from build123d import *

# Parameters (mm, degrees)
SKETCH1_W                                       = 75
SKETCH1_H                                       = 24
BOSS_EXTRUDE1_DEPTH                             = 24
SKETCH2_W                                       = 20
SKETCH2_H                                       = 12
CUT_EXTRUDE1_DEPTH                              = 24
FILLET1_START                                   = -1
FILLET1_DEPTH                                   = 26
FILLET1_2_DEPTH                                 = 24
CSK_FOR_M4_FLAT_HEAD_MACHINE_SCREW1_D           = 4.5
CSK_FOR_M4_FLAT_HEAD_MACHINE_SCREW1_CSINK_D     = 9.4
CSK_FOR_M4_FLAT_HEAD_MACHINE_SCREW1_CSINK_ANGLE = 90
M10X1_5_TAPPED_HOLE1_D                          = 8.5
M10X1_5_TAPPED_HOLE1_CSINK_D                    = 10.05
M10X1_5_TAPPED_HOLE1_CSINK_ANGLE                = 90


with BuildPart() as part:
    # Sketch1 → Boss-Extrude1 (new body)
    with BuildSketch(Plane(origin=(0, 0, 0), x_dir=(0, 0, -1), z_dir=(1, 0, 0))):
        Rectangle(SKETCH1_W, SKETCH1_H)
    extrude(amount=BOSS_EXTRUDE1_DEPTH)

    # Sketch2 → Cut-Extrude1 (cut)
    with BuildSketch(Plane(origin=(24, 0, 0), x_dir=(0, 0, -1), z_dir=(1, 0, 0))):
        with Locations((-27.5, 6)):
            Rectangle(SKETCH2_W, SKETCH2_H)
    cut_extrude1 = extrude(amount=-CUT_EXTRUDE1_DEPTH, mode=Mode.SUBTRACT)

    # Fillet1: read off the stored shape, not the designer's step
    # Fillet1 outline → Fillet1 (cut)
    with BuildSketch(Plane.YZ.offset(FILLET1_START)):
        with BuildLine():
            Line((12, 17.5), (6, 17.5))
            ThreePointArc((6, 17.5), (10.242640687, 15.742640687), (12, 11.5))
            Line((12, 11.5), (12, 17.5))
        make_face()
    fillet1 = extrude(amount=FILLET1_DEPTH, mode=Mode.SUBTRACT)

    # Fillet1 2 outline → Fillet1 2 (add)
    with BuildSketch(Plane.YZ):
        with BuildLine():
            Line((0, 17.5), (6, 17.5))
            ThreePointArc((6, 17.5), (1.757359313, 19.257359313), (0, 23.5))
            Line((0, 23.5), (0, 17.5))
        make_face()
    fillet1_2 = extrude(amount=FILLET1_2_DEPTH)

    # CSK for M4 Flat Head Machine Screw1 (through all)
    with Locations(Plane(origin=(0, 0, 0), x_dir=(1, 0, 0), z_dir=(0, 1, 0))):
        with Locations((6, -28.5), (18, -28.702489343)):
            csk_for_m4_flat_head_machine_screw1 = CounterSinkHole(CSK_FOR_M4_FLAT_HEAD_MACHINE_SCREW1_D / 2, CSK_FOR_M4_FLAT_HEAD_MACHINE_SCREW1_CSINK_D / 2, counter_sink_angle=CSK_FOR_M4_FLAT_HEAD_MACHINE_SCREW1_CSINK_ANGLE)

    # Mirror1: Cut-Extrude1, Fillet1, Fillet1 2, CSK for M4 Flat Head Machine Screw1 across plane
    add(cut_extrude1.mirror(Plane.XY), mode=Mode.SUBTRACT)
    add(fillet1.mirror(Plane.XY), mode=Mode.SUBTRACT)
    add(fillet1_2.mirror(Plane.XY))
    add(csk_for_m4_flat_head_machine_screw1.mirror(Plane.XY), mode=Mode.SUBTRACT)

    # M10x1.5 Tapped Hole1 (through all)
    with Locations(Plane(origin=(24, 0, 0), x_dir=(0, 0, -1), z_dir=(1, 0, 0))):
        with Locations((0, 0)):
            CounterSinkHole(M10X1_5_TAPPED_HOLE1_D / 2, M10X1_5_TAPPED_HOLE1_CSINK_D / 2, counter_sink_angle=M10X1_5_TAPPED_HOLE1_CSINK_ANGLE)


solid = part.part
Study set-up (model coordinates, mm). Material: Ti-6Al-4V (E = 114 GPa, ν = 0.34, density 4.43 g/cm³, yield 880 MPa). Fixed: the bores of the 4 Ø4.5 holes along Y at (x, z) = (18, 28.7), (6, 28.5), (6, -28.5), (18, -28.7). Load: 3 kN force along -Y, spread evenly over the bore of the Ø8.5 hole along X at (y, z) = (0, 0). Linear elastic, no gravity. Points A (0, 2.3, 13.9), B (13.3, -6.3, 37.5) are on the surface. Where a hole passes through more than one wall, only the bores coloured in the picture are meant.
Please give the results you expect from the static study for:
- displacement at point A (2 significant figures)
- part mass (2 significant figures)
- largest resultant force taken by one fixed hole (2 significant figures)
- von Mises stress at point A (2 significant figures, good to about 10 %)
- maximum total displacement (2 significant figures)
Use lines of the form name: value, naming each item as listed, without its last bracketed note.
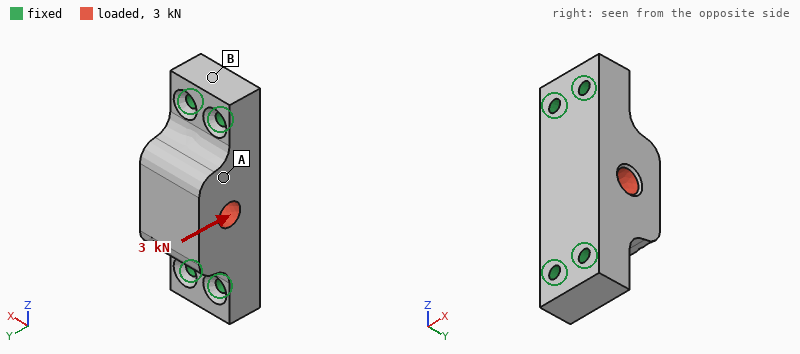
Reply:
displacement at point A: 3.4 µm
part mass: 130 g
largest resultant force taken by one fixed hole: 930 N
von Mises stress at point A: 9.0 MPa
maximum total displacement: 5.2 µm
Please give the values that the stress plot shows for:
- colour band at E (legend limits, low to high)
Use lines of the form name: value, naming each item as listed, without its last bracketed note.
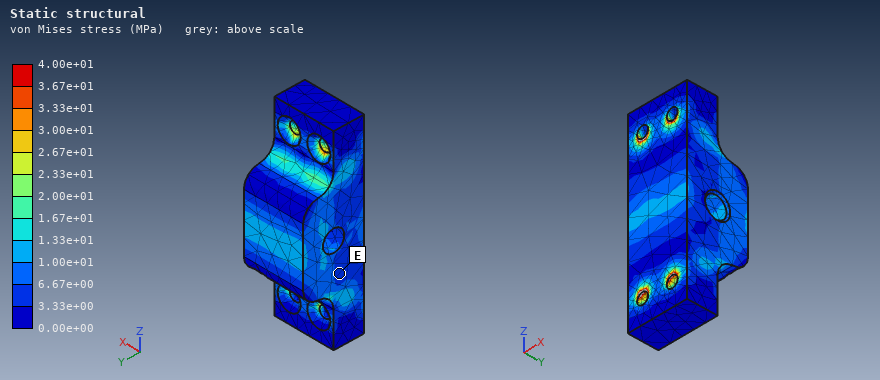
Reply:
colour band at E: 3.33e+00 to 6.67e+00 MPa
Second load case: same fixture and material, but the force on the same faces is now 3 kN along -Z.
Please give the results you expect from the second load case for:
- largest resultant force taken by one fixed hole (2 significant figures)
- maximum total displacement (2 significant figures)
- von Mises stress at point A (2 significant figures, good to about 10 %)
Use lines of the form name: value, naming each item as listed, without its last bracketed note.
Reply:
largest resultant force taken by one fixed hole: 790 N
maximum total displacement: 1.5 µm
von Mises stress at point A: 4.9 MPa
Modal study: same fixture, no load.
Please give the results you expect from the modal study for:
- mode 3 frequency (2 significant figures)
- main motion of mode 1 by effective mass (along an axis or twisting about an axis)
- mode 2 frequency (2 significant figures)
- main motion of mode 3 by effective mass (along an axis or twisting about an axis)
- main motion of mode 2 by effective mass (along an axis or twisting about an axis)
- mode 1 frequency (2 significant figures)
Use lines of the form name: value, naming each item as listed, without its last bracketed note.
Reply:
mode 3 frequency: 21 kHz
main motion of mode 1 by effective mass: along X
mode 2 frequency: 16 kHz
main motion of mode 3 by effective mass: along X
main motion of mode 2 by effective mass: along Y
mode 1 frequency: 12 kHz
